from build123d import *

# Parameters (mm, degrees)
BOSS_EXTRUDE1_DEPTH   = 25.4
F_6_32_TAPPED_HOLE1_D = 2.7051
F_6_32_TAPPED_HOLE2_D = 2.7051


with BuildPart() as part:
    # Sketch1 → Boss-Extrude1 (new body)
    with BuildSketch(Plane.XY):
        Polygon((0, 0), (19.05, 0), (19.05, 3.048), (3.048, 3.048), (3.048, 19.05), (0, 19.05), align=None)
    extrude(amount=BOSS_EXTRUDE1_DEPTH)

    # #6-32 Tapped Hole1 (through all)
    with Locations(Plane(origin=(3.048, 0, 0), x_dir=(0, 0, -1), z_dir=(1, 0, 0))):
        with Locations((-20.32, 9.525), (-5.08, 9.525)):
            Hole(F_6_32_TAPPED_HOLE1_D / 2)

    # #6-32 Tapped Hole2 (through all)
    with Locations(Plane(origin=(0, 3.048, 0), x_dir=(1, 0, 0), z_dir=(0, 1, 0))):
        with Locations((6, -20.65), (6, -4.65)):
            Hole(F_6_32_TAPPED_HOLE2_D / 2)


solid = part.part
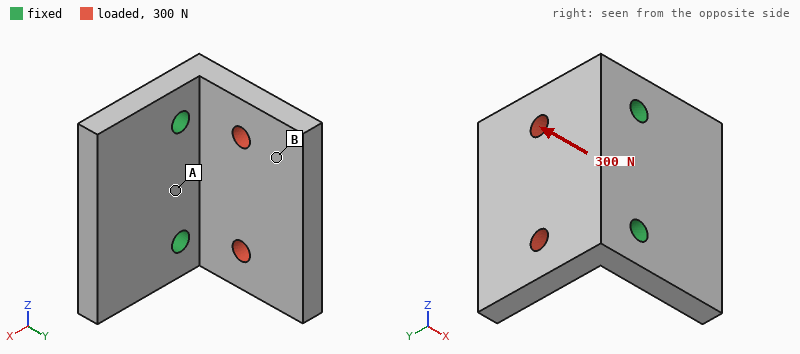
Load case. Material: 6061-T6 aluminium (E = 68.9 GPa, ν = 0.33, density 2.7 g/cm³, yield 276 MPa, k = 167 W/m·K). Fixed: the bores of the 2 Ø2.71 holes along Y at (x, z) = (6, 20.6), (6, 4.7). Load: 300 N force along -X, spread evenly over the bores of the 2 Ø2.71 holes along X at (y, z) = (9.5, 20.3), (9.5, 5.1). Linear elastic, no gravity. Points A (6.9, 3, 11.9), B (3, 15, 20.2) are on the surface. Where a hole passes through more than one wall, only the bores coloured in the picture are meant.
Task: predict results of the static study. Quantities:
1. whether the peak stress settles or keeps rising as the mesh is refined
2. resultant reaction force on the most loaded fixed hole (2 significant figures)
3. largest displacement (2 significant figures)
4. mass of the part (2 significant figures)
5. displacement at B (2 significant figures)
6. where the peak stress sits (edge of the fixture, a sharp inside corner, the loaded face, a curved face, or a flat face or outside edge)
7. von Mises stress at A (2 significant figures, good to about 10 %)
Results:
keeps rising
150 N
70 µm
7.1 g
51 µm
edge of the fixture
21 MPa
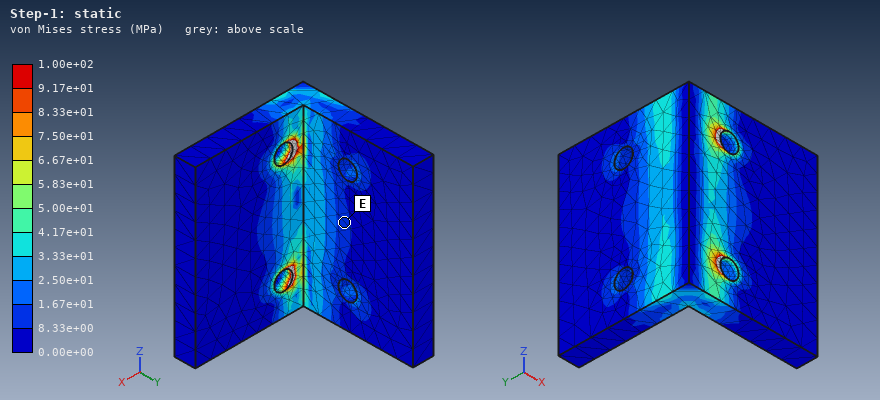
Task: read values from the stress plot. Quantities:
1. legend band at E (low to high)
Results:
8.33e+00 to 1.67e+01 MPa
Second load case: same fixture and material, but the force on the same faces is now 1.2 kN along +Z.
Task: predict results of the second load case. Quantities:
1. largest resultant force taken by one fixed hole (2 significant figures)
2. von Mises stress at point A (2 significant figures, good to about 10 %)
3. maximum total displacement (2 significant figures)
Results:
850 N
22 MPa
34 µm
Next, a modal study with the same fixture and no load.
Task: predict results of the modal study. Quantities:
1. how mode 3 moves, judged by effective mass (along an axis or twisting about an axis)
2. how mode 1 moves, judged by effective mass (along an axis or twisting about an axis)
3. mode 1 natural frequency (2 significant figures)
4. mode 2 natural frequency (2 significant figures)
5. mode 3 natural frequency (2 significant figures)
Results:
along Y
along X
6000 Hz
12 kHz
14 kHz
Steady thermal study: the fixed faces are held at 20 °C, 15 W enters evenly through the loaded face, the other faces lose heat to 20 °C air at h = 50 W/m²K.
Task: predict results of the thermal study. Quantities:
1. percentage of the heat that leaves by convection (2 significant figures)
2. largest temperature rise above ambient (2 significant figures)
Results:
4.6 %
16 K
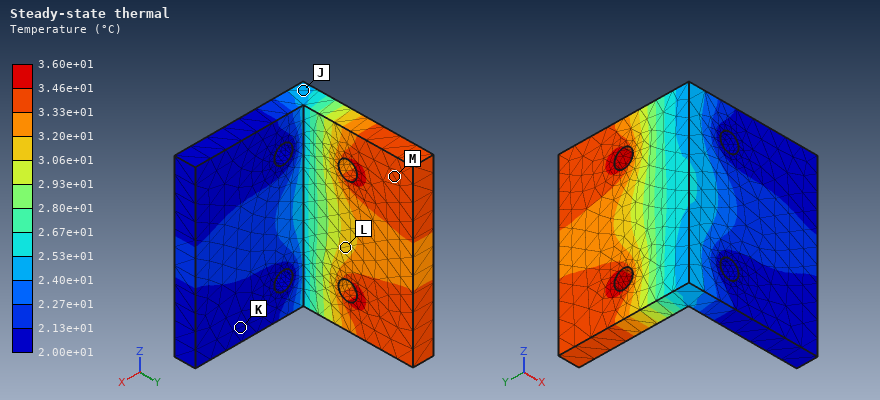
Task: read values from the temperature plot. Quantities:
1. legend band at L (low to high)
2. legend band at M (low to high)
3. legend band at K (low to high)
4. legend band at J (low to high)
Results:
3.06e+01 to 3.20e+01 °C
3.33e+01 to 3.46e+01 °C
2.00e+01 to 2.13e+01 °C
2.40e+01 to 2.53e+01 °C
